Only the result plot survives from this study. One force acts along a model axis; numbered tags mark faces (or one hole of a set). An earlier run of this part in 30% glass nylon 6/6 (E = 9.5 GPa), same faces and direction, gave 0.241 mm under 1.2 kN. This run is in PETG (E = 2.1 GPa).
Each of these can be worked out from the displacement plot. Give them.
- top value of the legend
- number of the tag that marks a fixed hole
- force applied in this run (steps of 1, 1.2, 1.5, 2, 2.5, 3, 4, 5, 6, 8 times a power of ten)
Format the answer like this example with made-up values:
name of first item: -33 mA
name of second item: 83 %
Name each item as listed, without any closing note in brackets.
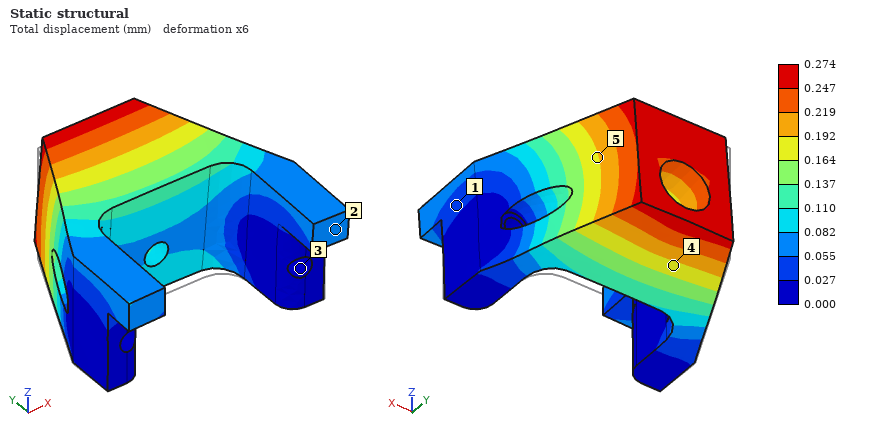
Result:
top value of the legend: 0.274 mm
number of the tag that marks a fixed hole: 3
force applied in this run: 300 N
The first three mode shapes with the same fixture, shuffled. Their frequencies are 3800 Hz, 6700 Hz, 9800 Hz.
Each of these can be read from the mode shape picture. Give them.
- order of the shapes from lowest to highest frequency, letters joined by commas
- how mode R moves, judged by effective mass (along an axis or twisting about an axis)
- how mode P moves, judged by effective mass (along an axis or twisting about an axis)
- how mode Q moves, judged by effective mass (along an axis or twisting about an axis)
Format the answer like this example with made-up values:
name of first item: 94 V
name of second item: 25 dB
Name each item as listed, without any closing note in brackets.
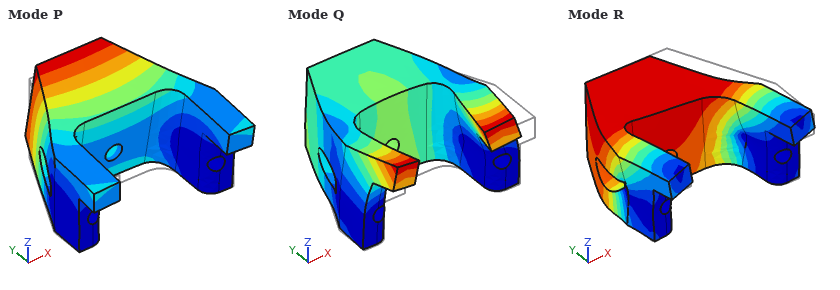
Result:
order of the shapes from lowest to highest frequency, letters joined by commas: P, R, Q
how mode R moves, judged by effective mass: along X
how mode P moves, judged by effective mass: along Z
how mode Q moves, judged by effective mass: along Y
